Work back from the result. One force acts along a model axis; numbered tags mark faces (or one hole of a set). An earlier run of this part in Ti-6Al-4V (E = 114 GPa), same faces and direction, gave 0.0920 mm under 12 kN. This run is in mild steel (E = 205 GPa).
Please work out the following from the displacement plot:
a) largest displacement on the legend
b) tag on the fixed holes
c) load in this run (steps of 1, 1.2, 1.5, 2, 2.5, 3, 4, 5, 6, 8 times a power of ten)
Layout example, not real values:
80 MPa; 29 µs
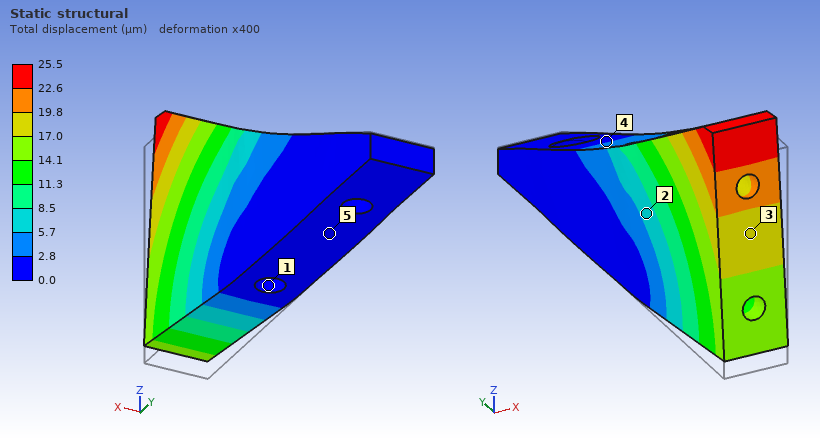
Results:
25.5 µm; 1; 6 kN
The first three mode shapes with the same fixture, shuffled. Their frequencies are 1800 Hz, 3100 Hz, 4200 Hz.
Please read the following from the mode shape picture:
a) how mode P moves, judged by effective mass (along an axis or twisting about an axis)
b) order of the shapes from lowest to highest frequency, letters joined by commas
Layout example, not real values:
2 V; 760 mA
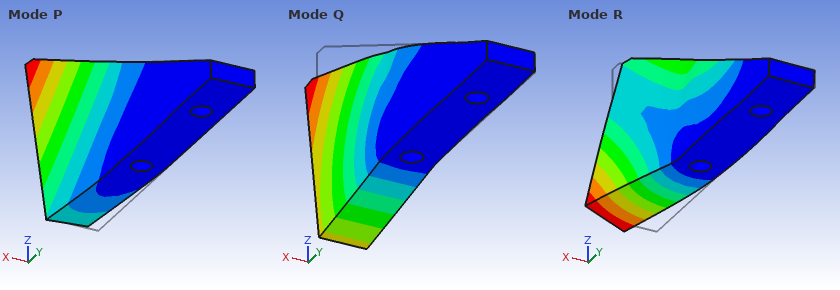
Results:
along X; P, Q, R
